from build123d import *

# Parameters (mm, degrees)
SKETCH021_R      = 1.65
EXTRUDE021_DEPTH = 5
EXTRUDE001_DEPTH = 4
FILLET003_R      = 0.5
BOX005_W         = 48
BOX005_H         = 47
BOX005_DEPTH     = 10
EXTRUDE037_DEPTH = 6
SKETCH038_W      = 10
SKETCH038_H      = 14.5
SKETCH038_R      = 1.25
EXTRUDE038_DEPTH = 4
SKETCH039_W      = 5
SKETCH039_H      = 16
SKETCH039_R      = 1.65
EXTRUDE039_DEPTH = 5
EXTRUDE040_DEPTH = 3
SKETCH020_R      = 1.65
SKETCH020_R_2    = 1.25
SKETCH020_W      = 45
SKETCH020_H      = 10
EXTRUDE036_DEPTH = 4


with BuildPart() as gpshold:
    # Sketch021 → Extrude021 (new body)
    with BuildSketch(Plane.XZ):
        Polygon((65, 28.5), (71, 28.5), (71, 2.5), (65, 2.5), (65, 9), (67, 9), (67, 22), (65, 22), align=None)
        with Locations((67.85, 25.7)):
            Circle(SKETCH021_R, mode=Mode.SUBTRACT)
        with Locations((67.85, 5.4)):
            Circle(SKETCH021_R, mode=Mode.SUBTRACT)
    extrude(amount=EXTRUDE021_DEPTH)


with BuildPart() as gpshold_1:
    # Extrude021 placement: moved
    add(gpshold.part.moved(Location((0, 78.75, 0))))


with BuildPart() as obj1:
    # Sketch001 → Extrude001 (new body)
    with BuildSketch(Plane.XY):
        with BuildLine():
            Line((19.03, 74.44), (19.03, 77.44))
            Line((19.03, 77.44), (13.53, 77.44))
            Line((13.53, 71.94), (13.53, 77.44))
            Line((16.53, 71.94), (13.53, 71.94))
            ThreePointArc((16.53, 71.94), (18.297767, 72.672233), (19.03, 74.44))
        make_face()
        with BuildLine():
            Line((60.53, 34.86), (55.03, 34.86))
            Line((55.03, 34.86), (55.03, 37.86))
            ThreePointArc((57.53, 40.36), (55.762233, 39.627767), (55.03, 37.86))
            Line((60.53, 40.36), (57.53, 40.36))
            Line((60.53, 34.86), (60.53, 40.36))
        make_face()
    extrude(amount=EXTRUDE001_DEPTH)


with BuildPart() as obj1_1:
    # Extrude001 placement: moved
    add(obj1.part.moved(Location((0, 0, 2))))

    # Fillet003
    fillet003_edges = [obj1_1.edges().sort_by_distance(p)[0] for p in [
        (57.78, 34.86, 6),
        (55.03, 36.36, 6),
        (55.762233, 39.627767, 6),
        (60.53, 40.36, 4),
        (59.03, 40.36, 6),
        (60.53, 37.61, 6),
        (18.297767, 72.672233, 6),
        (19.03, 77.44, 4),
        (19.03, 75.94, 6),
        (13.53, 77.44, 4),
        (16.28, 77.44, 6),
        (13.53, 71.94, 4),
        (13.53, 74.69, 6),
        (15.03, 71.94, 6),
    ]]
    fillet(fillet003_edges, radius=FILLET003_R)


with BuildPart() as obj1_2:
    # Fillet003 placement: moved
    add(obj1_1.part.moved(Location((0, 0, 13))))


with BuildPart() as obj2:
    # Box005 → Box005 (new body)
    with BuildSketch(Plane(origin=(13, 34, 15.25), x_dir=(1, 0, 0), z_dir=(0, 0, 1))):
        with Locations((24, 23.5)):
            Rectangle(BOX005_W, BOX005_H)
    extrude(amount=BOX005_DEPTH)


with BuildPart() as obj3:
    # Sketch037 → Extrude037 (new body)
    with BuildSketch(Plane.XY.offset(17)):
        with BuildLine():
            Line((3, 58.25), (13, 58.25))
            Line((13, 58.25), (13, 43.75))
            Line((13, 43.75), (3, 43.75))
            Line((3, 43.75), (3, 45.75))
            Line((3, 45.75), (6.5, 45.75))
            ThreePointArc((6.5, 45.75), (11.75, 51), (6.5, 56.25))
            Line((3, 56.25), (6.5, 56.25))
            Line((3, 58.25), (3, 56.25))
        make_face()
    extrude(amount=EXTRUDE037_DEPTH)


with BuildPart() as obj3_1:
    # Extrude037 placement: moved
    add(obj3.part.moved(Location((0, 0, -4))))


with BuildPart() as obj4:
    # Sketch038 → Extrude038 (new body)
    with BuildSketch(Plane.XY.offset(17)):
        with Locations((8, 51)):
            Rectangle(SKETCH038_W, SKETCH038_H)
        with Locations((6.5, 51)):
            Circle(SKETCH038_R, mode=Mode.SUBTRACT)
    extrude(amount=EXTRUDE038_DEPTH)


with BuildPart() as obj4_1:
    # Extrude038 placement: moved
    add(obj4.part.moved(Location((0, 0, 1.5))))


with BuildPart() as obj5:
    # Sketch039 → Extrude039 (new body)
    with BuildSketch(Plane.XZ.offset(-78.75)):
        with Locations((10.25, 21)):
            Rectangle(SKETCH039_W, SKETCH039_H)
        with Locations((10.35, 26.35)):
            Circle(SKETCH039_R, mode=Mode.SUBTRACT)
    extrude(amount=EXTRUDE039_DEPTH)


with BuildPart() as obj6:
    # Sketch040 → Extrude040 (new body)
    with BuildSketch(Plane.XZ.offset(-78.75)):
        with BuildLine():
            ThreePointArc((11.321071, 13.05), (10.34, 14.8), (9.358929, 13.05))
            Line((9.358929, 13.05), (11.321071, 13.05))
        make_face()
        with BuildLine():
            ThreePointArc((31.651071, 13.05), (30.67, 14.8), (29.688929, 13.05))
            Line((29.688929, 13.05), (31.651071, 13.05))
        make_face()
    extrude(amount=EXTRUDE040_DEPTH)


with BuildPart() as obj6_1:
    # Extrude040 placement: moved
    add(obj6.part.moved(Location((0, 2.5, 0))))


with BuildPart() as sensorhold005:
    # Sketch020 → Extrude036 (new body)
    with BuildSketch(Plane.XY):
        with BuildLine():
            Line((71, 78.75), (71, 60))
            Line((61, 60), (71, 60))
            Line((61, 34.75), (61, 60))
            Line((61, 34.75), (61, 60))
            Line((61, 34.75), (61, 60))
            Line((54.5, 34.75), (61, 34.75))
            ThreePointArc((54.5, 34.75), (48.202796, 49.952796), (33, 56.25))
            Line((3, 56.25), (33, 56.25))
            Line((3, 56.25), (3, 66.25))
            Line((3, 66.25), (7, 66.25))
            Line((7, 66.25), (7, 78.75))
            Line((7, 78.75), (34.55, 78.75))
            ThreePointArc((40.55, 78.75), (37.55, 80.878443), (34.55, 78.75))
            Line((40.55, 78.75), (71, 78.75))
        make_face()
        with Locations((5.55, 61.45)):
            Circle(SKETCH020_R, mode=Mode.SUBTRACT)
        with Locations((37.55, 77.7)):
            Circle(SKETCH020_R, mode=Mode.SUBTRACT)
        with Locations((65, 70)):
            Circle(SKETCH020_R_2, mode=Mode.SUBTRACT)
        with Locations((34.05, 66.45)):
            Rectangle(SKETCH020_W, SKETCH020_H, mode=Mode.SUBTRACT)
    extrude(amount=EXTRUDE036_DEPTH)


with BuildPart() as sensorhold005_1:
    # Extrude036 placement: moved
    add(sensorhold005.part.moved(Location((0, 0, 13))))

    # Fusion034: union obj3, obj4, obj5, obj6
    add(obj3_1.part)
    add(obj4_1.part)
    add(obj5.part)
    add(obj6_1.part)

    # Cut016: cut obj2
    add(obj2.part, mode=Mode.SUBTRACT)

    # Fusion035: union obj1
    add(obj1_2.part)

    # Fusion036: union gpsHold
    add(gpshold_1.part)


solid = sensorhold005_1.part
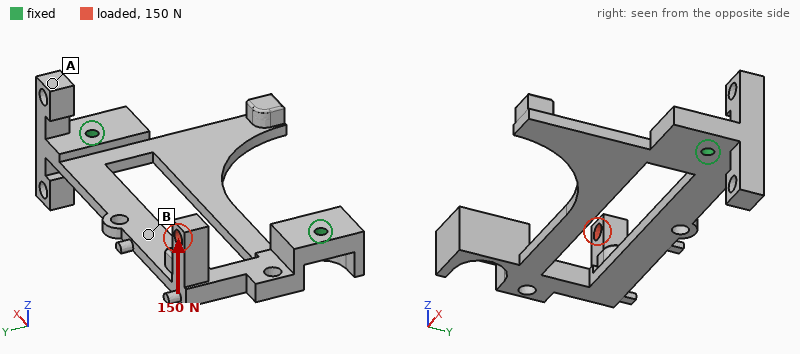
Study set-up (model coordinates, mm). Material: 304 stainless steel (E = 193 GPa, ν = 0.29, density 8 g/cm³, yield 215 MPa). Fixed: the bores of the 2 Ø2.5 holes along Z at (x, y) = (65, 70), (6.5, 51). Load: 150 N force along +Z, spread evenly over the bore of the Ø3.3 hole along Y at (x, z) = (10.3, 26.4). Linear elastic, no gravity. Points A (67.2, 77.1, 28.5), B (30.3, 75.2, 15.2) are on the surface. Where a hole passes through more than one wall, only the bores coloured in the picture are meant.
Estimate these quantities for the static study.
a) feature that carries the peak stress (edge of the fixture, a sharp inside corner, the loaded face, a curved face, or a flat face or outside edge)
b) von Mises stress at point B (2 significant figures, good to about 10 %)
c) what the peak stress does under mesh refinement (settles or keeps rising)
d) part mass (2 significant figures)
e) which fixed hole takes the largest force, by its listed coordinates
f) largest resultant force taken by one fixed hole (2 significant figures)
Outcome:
edge of the fixture
35 MPa
keeps rising
41 g
(6.5, 51)
160 N
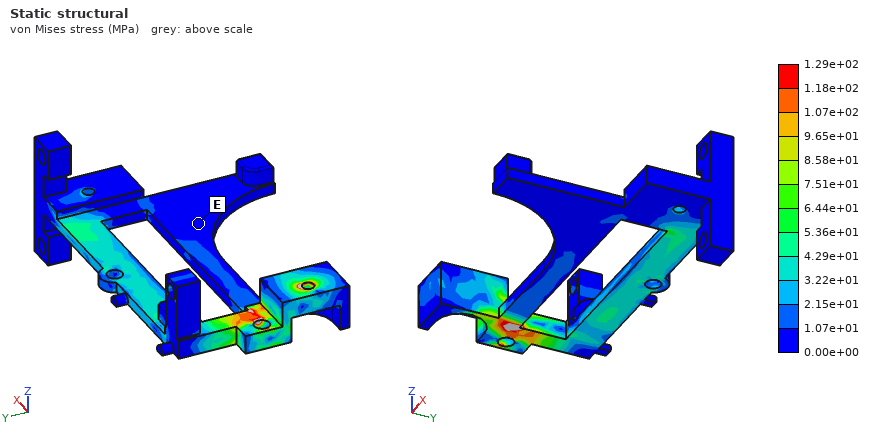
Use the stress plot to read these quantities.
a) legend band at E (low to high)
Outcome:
0.00e+00 to 1.07e+01 MPa
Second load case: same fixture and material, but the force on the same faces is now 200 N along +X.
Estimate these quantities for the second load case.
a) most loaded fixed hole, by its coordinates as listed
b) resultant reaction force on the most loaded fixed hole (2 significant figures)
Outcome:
(65, 70)
140 N
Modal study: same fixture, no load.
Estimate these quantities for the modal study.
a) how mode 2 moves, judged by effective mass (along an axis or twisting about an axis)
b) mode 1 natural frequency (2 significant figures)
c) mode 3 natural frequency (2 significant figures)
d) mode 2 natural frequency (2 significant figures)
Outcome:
along Z
1700 Hz
3900 Hz
2300 Hz
